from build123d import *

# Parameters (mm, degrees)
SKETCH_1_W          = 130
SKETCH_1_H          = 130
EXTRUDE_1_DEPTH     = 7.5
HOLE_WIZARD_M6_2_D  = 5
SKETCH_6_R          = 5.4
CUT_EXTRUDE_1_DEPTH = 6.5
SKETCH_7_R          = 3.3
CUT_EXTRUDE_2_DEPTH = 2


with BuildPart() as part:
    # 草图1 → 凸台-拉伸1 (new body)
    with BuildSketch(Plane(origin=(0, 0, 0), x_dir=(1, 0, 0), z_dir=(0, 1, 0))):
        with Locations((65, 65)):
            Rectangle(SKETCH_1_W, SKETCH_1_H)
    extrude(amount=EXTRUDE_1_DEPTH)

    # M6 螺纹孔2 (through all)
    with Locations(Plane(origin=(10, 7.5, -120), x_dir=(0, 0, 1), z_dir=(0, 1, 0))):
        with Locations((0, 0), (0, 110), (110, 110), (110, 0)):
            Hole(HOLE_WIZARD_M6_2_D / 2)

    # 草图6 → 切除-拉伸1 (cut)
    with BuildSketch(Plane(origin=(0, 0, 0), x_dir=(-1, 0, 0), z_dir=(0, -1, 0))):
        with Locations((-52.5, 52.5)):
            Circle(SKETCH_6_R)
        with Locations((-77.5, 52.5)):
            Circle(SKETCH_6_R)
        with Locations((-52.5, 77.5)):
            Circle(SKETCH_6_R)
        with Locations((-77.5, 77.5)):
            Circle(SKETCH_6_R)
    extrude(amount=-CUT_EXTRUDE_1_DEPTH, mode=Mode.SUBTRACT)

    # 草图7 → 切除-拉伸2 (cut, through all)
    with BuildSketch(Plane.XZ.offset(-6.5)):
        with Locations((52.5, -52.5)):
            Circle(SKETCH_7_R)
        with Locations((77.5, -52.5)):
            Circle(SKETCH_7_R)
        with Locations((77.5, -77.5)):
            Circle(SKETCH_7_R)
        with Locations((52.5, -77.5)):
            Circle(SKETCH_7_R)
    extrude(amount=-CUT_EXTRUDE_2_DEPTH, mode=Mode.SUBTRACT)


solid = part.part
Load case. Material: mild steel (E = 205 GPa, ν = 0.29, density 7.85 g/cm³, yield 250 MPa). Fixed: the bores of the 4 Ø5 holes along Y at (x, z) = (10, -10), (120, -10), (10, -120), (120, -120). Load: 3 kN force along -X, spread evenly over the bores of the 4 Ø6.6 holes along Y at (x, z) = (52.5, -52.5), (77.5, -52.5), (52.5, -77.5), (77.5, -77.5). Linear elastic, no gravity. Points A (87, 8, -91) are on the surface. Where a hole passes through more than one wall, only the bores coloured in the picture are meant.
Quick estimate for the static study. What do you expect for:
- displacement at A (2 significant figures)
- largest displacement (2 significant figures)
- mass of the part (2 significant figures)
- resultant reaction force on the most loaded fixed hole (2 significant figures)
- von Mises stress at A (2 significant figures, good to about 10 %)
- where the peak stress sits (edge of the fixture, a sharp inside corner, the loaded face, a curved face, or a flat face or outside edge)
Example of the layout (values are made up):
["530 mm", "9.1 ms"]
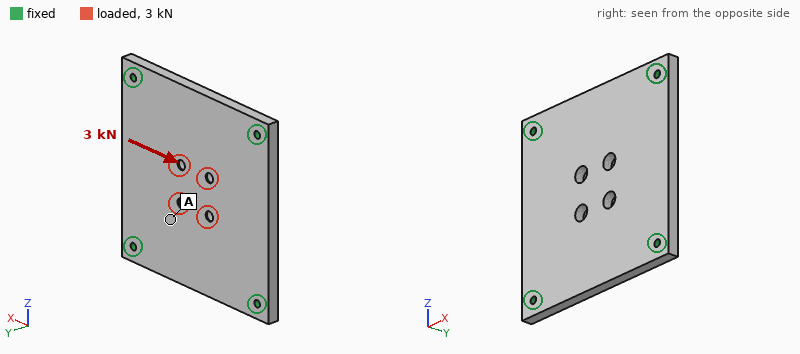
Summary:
["1.6 µm", "3.0 µm", "970 g", "840 N", "5.2 MPa", "the loaded face"]
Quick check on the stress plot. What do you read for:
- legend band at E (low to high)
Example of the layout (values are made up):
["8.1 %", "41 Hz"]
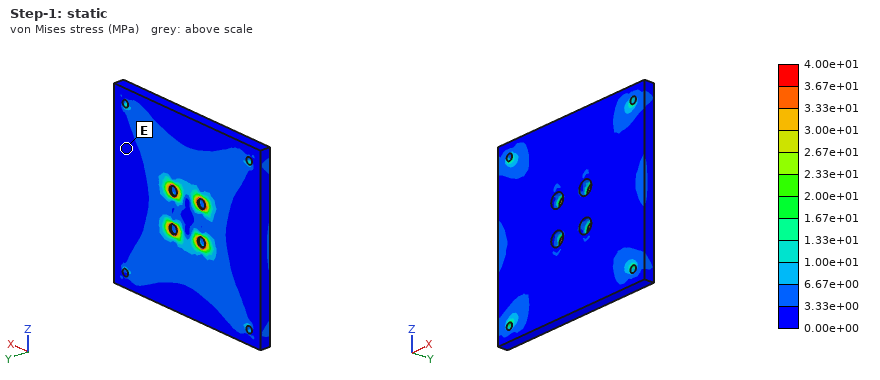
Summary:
["0.00e+00 to 3.33e+00 MPa"]
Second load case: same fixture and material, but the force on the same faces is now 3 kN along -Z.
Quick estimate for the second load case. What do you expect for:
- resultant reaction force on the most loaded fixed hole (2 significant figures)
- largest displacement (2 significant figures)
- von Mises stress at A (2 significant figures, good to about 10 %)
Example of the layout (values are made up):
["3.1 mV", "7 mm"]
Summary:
["840 N", "3.0 µm", "5.2 MPa"]
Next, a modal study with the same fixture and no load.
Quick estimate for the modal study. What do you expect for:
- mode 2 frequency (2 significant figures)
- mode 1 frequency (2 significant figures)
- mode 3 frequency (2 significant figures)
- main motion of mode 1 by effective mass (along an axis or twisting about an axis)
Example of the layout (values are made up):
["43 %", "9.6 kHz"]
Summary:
["3300 Hz", "2000 Hz", "3300 Hz", "along Y"]
